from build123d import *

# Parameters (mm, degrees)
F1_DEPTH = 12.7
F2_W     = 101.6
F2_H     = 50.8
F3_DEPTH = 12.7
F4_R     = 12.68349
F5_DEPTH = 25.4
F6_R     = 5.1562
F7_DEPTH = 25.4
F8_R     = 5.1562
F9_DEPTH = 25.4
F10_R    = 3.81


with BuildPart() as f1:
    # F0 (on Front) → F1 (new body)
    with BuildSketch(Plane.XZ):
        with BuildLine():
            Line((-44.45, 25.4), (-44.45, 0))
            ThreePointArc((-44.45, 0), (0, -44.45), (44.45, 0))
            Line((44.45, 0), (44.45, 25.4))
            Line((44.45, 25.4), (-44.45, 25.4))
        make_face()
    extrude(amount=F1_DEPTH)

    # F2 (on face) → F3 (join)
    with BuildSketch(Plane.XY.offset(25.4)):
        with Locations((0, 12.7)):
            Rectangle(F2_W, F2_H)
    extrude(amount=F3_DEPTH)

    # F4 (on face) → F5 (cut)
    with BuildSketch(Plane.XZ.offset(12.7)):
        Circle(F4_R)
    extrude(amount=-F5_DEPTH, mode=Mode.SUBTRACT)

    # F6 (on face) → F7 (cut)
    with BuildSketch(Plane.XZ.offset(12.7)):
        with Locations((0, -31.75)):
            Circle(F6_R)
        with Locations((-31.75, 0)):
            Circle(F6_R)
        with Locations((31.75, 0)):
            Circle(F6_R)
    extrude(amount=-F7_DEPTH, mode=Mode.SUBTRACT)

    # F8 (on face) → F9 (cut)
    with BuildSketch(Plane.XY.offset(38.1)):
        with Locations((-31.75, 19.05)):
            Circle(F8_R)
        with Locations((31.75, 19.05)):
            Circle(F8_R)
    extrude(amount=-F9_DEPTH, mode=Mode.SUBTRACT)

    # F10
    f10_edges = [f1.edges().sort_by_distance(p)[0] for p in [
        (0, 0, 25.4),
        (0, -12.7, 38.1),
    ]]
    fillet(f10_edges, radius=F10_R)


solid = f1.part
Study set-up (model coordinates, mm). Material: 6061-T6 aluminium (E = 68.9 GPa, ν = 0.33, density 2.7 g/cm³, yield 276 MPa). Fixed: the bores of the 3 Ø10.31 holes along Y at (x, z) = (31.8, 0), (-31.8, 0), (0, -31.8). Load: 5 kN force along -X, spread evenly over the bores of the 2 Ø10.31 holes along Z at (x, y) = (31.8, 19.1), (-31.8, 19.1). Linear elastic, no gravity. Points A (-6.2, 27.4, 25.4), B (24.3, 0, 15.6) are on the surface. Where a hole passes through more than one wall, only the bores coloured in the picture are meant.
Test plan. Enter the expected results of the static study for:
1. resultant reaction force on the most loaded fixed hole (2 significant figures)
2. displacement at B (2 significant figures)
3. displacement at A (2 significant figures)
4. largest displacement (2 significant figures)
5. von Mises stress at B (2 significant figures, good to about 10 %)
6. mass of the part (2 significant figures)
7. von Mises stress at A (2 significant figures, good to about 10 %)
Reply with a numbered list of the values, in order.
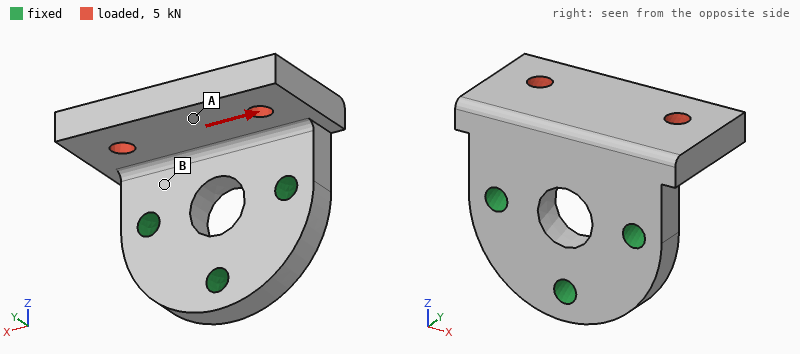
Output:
1. 3.8 kN
2. 9.4 µm
3. 37 µm
4. 60 µm
5. 23 MPa
6. 330 g
7. 7.8 MPa
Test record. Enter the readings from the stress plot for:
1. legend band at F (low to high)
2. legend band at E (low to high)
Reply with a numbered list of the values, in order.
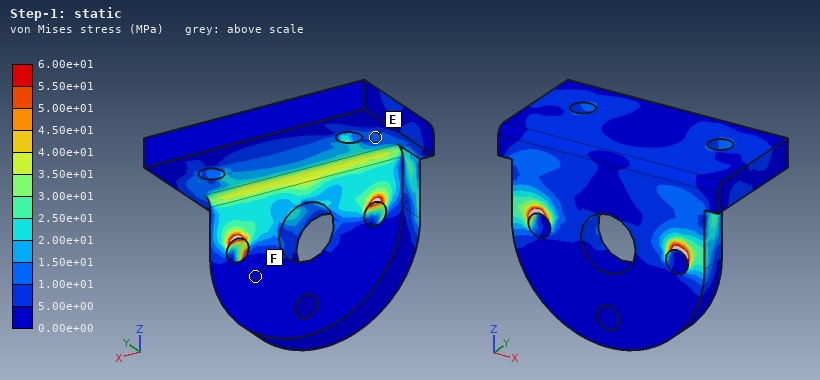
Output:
1. 0.00e+00 to 5.00e+00 MPa
2. 1.00e+01 to 1.50e+01 MPa
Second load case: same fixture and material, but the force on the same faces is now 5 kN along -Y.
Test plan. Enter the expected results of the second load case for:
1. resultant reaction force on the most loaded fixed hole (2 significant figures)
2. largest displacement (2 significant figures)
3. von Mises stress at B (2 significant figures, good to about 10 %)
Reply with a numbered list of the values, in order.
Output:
1. 2.8 kN
2. 0.15 mm
3. 38 MPa
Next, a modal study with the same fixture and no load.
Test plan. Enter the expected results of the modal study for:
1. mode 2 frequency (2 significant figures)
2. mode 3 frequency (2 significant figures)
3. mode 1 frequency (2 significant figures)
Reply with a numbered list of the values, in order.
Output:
1. 3700 Hz
2. 6300 Hz
3. 2200 Hz
